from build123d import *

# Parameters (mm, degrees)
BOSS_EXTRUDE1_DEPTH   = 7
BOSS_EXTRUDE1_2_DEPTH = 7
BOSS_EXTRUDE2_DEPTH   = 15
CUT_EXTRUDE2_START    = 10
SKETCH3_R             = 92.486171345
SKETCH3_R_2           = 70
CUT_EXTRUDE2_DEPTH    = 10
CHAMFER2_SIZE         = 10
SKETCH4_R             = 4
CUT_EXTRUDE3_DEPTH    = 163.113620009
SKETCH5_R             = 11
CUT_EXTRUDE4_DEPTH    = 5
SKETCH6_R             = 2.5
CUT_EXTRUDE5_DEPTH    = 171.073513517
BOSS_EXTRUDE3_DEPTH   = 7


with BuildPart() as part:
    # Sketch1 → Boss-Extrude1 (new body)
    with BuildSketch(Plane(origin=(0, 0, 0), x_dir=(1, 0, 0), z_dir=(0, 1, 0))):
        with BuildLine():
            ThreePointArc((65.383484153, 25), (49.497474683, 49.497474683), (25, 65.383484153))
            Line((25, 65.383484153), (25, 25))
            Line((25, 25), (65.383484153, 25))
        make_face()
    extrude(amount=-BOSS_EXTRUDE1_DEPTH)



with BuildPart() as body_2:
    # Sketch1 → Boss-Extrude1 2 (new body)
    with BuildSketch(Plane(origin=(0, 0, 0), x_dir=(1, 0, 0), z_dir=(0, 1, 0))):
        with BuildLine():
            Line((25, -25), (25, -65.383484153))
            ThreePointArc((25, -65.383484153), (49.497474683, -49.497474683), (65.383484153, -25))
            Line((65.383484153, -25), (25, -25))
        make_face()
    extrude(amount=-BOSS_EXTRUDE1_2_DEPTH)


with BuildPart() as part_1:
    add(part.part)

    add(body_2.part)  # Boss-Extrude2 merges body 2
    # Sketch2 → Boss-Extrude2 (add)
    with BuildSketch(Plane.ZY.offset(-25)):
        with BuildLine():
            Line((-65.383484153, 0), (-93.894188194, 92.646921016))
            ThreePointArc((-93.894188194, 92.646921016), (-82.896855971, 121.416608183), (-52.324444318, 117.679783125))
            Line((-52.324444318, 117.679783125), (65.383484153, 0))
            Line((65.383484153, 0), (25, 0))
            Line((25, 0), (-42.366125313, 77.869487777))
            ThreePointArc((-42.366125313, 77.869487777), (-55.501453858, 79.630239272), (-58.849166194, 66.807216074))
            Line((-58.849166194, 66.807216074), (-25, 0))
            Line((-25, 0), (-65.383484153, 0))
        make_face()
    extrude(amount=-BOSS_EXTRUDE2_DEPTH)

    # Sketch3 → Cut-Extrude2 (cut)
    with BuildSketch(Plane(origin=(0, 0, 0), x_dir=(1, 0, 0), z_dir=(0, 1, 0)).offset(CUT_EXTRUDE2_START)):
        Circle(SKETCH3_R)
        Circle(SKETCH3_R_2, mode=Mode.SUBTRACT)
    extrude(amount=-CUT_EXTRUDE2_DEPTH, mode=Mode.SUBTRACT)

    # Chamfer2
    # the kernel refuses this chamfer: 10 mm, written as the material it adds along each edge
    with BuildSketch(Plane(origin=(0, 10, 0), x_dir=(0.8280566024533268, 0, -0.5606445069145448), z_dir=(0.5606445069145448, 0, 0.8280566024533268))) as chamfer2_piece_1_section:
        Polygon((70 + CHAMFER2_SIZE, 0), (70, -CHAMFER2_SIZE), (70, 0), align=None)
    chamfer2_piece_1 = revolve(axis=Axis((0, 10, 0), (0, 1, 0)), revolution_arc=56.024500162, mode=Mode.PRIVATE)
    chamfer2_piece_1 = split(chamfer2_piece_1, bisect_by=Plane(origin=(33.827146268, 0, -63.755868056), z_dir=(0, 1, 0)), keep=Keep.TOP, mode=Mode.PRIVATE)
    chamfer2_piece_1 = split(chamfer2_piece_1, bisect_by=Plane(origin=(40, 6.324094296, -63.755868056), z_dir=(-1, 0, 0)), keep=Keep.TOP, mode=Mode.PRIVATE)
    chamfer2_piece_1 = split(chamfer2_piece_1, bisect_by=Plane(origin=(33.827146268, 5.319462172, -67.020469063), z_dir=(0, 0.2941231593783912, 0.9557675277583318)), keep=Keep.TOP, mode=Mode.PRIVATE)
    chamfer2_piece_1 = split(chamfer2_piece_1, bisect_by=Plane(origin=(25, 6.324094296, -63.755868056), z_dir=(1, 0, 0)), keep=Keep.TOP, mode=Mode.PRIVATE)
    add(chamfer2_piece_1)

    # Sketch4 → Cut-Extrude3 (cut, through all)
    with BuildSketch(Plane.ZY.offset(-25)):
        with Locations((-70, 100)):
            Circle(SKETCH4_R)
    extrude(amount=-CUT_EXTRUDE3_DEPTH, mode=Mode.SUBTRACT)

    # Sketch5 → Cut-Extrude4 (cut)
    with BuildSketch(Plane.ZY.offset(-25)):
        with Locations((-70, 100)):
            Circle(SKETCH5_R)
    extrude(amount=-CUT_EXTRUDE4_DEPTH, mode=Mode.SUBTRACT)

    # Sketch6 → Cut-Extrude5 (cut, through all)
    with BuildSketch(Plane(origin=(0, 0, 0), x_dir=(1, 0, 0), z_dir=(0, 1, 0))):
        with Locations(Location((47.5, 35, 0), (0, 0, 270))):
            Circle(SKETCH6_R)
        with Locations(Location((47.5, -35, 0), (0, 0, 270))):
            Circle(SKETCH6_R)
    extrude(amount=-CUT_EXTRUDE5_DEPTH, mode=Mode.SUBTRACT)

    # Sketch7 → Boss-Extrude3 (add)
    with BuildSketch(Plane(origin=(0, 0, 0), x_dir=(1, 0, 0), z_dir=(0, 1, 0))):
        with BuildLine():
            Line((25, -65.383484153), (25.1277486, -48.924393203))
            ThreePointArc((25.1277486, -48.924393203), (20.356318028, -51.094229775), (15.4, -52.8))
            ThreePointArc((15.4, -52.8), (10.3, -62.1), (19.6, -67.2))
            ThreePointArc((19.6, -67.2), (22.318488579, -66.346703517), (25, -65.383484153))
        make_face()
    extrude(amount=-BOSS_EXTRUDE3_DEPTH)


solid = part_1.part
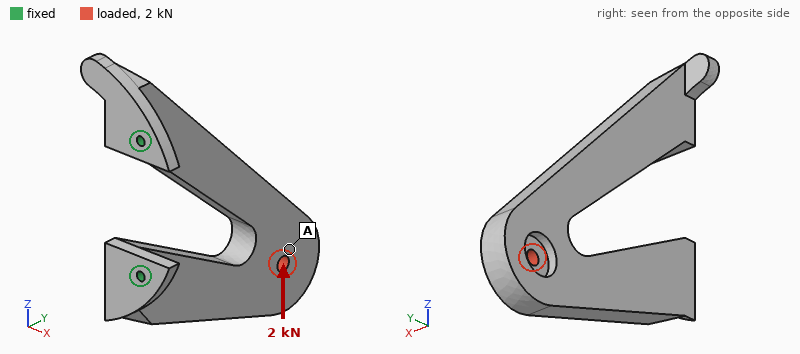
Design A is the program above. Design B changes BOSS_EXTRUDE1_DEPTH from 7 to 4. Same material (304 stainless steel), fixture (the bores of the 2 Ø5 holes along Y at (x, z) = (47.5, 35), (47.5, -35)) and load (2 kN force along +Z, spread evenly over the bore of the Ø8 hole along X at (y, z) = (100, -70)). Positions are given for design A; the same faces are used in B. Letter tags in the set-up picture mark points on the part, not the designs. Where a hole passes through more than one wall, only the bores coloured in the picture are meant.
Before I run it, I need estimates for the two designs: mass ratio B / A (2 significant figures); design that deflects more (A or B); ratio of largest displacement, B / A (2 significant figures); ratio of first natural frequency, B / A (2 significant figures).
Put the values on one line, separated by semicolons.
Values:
0.98; B; 1.6; 0.76
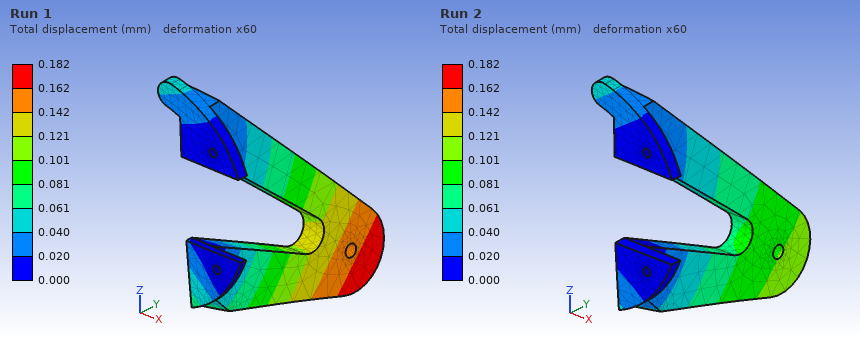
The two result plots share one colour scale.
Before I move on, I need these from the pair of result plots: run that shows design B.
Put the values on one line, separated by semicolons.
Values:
Run 1
